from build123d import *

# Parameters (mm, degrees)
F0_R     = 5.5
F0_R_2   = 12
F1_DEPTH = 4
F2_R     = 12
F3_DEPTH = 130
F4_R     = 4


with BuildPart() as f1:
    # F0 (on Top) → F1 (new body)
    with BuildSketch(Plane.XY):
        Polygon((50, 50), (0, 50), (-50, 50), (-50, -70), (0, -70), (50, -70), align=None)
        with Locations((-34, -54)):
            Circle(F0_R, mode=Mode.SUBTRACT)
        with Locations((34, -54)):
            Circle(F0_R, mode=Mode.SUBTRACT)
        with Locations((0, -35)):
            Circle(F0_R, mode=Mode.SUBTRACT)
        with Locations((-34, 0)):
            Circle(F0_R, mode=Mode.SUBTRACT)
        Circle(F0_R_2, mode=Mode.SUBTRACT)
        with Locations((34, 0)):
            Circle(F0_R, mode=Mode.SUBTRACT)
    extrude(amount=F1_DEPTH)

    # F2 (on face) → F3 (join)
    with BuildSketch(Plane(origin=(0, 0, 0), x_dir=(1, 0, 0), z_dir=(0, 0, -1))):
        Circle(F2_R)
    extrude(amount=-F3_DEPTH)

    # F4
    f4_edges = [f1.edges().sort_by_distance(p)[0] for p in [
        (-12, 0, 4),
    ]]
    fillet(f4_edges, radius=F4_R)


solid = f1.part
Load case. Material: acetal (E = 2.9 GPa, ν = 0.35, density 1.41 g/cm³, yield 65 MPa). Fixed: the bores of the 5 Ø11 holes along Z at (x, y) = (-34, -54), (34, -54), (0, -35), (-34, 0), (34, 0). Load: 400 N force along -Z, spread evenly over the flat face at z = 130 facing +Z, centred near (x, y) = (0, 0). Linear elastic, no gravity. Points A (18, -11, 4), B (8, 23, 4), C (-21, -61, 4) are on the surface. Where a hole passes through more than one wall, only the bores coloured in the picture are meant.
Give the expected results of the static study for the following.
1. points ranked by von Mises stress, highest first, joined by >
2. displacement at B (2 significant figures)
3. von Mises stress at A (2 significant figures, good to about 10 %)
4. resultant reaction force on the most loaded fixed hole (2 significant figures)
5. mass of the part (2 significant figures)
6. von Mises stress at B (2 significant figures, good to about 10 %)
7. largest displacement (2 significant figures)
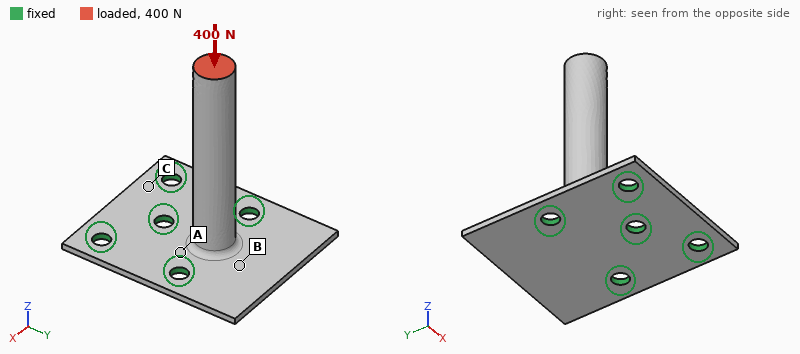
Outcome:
A > B > C
0.34 mm
4.6 MPa
180 N
150 g
3.5 MPa
0.90 mm
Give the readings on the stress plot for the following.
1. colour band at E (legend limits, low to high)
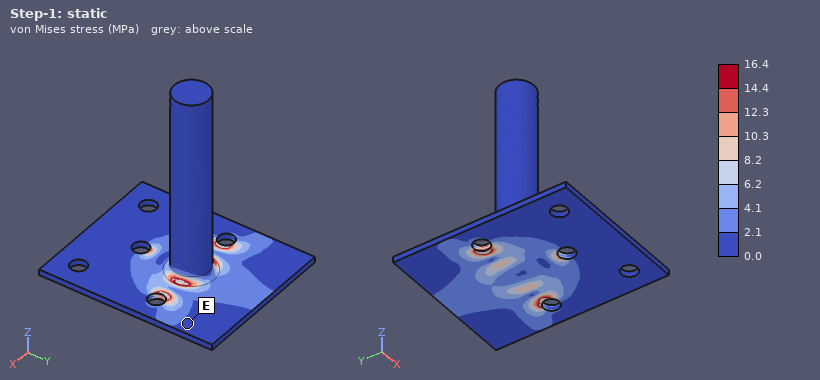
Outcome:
0.0 to 2.1 MPa
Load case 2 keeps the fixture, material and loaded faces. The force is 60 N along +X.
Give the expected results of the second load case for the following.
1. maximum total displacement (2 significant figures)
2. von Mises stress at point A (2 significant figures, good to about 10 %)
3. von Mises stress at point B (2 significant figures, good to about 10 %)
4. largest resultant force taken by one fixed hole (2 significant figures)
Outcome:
2.2 mm
5.4 MPa
2.8 MPa
160 N
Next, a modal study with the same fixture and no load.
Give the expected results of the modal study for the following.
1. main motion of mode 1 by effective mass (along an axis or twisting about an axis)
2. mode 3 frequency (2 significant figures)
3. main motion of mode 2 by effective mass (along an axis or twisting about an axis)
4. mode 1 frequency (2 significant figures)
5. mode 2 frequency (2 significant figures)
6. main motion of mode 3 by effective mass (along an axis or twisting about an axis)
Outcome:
along Y
490 Hz
along X
130 Hz
170 Hz
along Z
